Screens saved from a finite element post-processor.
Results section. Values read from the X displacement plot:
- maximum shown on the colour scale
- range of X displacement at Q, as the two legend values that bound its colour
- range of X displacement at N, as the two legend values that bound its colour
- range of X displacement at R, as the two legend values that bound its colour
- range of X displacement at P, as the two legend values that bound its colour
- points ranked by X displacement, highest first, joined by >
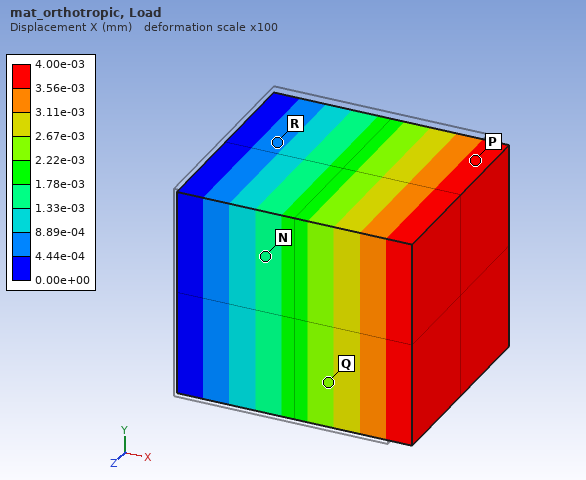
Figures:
4.00e-03 mm
2.22e-03 to 2.67e-03 mm
1.33e-03 to 1.78e-03 mm
4.44e-04 to 8.89e-04 mm
3.56e-03 to 4.00e-03 mm
P > Q > N > R
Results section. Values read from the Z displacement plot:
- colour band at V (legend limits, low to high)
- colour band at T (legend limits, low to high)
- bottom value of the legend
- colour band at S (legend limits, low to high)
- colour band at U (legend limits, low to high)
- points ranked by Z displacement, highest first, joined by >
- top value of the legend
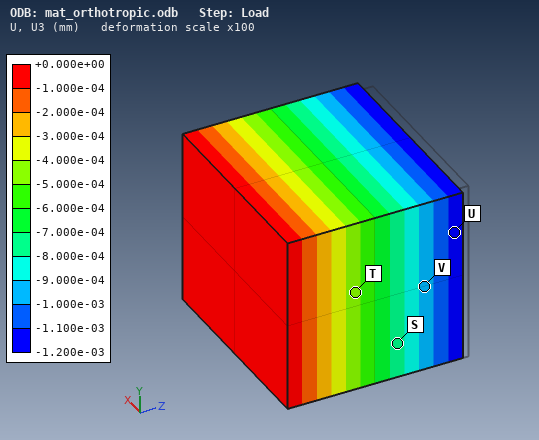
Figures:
-1.000e-03 to -9.000e-04 mm
-5.000e-04 to -4.000e-04 mm
-1.200e-03 mm
-8.000e-04 to -7.000e-04 mm
-1.200e-03 to -1.100e-03 mm
T > S > V > U
+0.000e+00 mm
